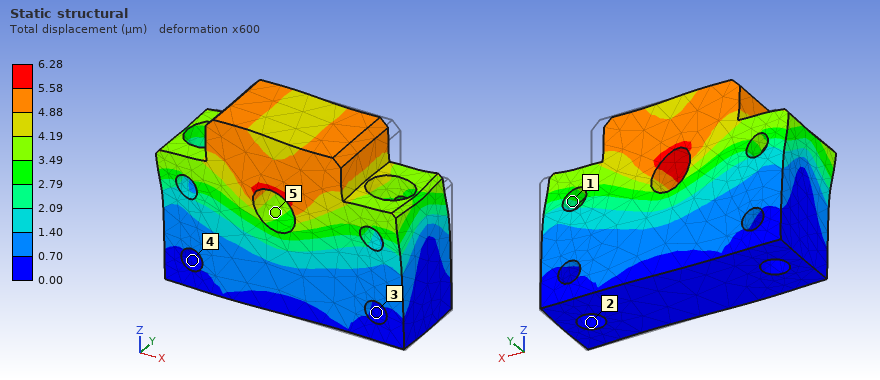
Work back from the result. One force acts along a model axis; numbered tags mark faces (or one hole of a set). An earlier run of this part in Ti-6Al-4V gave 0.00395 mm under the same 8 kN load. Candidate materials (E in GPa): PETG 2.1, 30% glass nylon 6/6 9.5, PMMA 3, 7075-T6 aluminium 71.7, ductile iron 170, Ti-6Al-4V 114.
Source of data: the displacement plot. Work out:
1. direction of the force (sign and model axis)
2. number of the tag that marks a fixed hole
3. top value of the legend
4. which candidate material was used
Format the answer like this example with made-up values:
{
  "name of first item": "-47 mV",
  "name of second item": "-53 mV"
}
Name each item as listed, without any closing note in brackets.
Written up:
{
  "direction of the force": "-X",
  "number of the tag that marks a fixed hole": "2",
  "top value of the legend": "6.28 µm",
  "which candidate material was used": "7075-T6 aluminium"
}
